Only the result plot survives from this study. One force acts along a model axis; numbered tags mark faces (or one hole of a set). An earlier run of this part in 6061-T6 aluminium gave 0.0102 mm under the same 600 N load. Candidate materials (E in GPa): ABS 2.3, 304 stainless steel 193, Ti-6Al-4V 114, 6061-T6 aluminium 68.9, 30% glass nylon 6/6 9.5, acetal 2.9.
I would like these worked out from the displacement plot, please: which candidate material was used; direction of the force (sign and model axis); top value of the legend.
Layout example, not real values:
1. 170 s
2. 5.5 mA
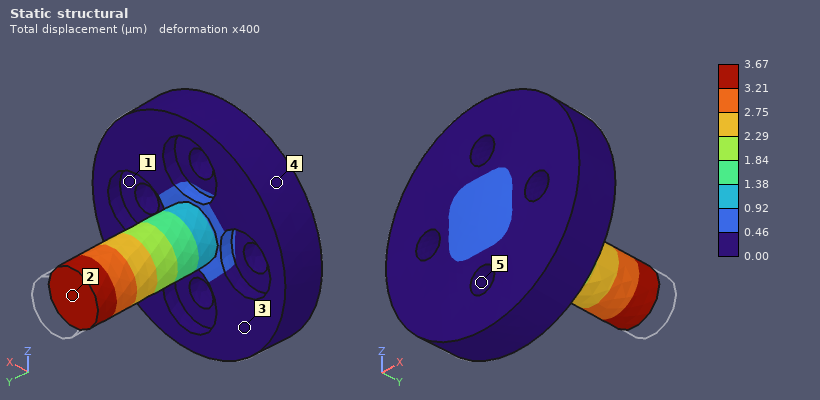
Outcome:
1. 304 stainless steel
2. -Y
3. 3.67 µm
